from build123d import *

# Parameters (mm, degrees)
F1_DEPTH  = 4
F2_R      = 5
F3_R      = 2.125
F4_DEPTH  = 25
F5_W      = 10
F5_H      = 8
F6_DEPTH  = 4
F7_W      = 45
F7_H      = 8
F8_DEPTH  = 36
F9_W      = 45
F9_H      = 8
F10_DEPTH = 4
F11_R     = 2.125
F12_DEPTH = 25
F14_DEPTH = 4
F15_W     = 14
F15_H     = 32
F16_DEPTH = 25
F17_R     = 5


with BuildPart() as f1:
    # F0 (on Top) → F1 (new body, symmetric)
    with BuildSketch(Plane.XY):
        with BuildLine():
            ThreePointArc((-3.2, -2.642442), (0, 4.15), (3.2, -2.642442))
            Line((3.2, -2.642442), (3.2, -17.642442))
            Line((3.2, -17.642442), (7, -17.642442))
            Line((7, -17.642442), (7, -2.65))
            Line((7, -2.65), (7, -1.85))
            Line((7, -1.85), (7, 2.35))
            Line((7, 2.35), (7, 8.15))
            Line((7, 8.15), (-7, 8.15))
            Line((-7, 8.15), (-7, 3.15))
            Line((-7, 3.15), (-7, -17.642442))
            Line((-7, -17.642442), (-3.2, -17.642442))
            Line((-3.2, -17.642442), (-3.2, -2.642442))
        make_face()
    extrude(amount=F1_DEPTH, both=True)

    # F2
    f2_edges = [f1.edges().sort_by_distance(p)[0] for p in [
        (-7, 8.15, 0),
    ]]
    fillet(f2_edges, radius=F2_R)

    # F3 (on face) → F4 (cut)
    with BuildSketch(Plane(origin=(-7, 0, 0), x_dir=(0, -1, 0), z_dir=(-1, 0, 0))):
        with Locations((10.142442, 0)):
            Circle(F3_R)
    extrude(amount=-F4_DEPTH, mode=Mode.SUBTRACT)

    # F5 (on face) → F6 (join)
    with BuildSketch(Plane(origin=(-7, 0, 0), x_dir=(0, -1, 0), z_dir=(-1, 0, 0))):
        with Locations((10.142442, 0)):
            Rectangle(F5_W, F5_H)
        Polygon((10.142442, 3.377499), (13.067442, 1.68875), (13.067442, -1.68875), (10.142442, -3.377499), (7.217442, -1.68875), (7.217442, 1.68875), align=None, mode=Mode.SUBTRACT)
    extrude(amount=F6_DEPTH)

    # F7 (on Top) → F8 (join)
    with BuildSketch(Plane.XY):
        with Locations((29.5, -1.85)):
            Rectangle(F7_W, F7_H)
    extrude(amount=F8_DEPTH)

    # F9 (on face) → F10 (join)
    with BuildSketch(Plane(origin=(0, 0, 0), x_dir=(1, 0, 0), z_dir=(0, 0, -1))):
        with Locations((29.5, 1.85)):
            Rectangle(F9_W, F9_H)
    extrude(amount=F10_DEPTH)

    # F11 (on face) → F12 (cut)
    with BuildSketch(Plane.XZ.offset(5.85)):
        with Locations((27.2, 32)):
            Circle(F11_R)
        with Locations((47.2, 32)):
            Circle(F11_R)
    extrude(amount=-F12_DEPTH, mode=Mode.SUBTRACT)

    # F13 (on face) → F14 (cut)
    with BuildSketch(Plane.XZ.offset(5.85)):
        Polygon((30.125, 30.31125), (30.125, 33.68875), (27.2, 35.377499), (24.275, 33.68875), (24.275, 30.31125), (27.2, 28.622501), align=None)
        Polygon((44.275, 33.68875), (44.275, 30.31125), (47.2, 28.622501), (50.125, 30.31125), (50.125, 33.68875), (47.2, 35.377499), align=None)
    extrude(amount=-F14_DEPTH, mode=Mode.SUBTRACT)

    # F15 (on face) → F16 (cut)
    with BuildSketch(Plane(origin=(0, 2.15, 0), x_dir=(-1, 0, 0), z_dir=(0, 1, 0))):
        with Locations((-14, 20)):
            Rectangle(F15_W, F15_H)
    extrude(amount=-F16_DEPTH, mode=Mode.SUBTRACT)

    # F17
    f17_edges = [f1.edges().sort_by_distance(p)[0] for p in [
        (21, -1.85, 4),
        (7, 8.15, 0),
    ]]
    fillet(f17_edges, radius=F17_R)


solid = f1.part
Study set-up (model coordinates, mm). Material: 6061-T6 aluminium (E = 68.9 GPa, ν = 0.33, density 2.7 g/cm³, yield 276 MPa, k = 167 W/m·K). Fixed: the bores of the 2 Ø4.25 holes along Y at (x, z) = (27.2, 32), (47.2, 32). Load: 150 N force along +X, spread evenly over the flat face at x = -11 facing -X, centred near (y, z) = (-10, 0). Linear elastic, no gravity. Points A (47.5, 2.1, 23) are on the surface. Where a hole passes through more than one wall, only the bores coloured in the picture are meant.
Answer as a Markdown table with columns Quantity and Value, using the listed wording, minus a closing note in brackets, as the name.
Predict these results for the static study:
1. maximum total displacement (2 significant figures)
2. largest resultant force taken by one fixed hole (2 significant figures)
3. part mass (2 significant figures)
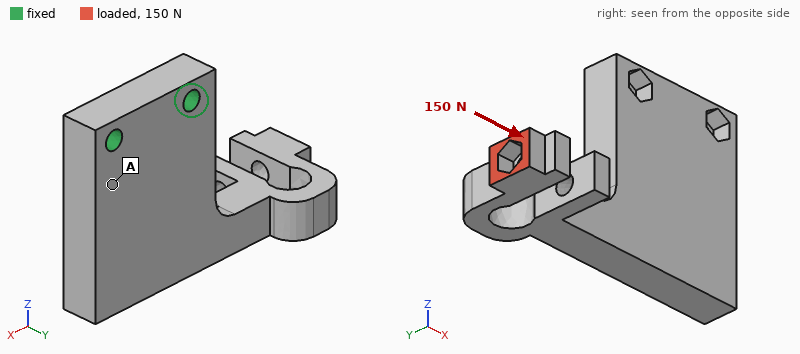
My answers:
| Quantity | Value |
|---|---|
| maximum total displacement | 0.44 mm |
| largest resultant force taken by one fixed hole | 240 N |
| part mass | 33 g |
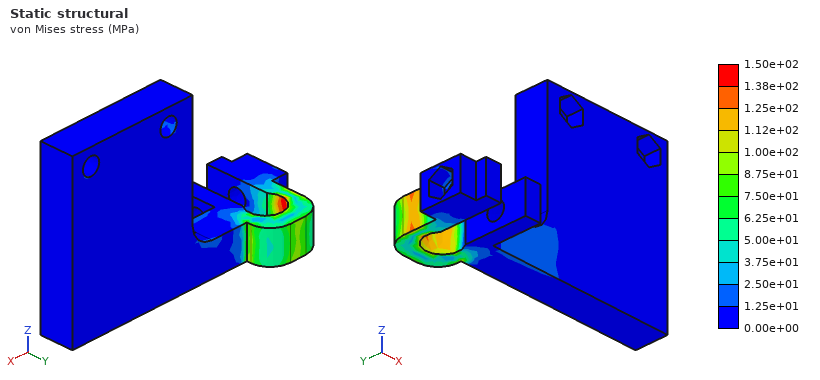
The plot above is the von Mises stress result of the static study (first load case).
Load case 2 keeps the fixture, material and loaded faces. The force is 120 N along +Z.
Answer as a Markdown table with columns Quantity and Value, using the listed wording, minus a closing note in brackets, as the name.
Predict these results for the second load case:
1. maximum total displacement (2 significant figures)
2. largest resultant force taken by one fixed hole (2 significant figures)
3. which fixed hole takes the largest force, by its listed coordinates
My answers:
| Quantity | Value |
|---|---|
| maximum total displacement | 0.32 mm |
| largest resultant force taken by one fixed hole | 320 N |
| which fixed hole takes the largest force, by its listed coordinates | (27.2, 32) |
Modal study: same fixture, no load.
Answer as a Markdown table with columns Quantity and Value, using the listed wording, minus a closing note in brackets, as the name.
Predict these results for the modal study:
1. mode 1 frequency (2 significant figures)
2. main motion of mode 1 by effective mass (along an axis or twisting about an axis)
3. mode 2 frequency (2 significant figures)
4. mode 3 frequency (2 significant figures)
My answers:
| Quantity | Value |
|---|---|
| mode 1 frequency | 1900 Hz |
| main motion of mode 1 by effective mass | along Y |
| mode 2 frequency | 2600 Hz |
| mode 3 frequency | 2900 Hz |
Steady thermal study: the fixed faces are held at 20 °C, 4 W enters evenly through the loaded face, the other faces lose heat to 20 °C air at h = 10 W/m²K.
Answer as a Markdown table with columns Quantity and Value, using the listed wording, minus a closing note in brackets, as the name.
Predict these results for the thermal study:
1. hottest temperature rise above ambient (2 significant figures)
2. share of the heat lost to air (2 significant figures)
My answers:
| Quantity | Value |
|---|---|
| hottest temperature rise above ambient | 33 K |
| share of the heat lost to air | 9.8 % |
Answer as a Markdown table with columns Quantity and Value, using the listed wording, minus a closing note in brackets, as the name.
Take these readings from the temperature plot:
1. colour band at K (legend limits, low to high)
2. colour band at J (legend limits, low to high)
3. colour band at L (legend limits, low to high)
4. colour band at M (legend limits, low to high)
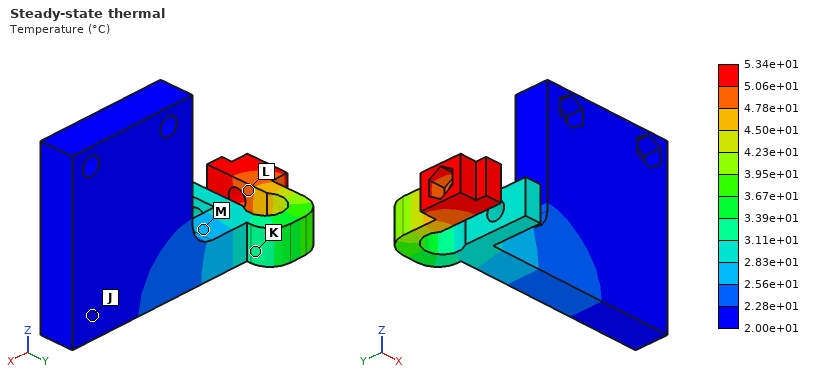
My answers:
| Quantity | Value |
|---|---|
| colour band at K | 3.11e+01 to 3.39e+01 °C |
| colour band at J | 2.00e+01 to 2.28e+01 °C |
| colour band at L | 4.78e+01 to 5.06e+01 °C |
| colour band at M | 2.56e+01 to 2.83e+01 °C |
